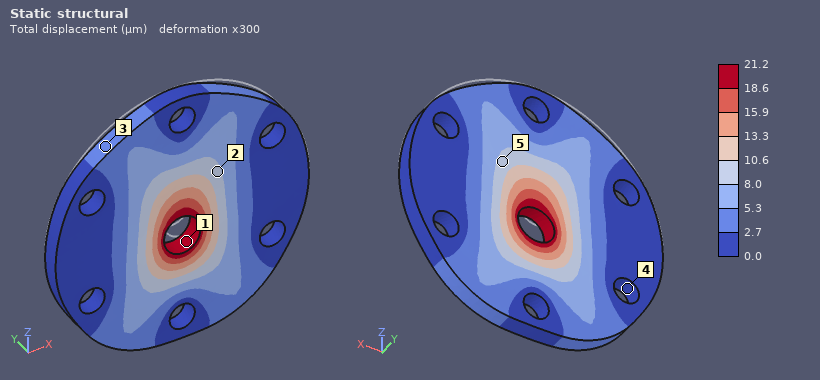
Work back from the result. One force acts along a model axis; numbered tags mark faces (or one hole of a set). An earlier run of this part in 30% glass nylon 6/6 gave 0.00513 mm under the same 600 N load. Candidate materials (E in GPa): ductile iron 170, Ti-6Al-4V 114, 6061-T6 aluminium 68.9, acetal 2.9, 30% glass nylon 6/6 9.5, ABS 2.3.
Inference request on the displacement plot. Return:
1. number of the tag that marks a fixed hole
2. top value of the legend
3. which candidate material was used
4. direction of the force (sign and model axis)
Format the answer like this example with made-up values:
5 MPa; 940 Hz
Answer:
4; 21.2 µm; ABS; -Z
